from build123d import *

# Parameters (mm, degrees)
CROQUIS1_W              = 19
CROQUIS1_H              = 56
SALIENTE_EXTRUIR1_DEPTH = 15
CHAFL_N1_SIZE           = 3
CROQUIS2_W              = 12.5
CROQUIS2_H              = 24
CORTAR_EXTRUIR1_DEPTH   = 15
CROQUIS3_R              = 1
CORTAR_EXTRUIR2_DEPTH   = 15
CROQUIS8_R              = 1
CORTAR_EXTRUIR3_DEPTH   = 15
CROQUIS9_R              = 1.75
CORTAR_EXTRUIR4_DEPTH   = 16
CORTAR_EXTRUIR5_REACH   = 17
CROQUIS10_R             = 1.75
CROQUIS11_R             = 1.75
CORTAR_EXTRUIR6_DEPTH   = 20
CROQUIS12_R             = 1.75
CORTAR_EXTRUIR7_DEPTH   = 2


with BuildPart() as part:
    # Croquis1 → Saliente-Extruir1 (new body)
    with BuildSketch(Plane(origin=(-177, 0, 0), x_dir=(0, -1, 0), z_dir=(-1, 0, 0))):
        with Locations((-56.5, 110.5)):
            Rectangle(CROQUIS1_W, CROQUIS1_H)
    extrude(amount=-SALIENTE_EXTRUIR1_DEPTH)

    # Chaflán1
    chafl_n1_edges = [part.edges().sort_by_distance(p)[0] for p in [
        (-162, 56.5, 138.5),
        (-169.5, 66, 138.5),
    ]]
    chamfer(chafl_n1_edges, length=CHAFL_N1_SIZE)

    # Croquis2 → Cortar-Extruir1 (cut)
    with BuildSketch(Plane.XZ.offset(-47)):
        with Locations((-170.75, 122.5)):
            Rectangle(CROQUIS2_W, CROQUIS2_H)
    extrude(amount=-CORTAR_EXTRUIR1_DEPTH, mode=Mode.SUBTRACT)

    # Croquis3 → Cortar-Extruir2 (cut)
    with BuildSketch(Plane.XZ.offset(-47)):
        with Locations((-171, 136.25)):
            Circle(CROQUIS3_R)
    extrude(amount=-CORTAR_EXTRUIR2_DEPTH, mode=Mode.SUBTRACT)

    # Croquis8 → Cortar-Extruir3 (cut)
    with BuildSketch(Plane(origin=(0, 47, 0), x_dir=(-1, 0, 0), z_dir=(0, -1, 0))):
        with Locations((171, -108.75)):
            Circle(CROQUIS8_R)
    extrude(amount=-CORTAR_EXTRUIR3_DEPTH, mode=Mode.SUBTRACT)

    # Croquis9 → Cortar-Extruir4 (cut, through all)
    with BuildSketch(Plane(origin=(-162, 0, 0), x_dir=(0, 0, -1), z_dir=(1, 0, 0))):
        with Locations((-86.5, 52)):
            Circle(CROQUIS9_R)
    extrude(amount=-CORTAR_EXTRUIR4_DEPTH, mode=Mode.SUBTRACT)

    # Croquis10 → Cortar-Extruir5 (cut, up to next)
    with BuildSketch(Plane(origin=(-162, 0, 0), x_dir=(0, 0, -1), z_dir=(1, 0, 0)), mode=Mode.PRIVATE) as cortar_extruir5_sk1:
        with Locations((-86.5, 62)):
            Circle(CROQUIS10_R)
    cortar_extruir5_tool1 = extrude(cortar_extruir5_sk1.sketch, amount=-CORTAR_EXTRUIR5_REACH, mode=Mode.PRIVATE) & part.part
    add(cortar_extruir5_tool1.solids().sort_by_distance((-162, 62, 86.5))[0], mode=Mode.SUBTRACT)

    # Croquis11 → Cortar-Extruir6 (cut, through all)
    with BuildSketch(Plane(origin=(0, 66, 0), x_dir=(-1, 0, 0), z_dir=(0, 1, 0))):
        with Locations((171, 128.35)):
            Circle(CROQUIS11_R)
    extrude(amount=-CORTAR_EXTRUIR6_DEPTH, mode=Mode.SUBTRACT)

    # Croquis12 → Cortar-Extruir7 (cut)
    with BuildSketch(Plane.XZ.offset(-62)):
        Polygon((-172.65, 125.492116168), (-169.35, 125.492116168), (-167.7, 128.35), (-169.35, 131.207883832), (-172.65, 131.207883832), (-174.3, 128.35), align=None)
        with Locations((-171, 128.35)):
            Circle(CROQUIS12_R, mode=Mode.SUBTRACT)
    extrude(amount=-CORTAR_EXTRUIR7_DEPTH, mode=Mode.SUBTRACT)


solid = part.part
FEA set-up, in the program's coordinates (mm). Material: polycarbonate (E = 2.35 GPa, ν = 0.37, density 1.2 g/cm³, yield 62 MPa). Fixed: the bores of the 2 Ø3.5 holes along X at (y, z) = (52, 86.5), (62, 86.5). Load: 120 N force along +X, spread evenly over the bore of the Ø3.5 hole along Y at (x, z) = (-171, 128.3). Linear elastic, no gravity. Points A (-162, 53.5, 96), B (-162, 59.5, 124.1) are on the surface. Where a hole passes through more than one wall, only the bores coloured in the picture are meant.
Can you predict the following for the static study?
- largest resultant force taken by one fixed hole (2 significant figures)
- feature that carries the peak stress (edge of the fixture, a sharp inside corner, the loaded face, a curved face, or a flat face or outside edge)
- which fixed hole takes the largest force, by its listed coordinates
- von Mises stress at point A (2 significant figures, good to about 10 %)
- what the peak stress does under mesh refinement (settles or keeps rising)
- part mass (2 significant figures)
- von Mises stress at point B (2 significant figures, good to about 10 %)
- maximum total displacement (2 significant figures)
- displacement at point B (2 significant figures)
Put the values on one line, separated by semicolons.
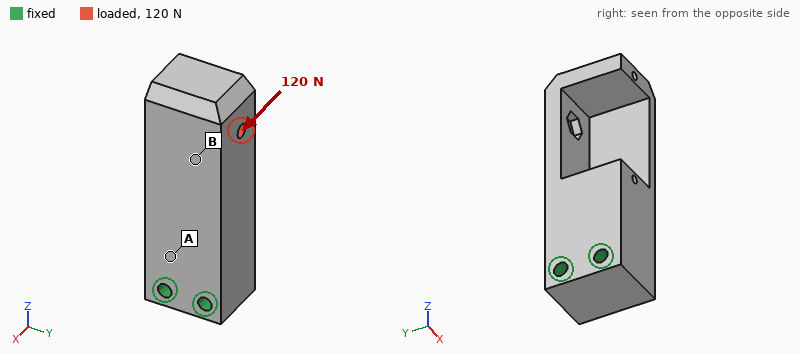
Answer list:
98 N; a sharp inside corner; (62, 86.5); 5.4 MPa; keeps rising; 13 g; 2.3 MPa; 0.64 mm; 0.34 mm
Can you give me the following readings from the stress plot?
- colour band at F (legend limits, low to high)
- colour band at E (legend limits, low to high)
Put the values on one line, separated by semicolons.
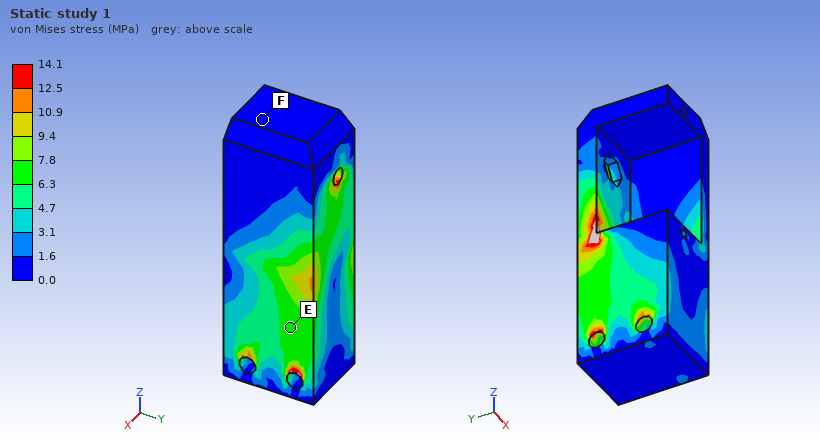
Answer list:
0.0 to 1.6 MPa; 6.3 to 7.8 MPa
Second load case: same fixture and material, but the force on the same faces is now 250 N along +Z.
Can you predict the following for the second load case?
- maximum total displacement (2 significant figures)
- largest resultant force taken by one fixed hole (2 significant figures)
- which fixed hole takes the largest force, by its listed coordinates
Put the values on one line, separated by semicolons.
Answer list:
0.27 mm; 290 N; (62, 86.5)
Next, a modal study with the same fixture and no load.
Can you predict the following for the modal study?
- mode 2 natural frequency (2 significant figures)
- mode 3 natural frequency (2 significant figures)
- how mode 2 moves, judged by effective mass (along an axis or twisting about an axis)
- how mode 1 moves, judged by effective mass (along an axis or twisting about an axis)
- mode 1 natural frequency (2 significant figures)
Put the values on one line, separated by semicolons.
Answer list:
1400 Hz; 2500 Hz; along Y; along X; 1100 Hz
